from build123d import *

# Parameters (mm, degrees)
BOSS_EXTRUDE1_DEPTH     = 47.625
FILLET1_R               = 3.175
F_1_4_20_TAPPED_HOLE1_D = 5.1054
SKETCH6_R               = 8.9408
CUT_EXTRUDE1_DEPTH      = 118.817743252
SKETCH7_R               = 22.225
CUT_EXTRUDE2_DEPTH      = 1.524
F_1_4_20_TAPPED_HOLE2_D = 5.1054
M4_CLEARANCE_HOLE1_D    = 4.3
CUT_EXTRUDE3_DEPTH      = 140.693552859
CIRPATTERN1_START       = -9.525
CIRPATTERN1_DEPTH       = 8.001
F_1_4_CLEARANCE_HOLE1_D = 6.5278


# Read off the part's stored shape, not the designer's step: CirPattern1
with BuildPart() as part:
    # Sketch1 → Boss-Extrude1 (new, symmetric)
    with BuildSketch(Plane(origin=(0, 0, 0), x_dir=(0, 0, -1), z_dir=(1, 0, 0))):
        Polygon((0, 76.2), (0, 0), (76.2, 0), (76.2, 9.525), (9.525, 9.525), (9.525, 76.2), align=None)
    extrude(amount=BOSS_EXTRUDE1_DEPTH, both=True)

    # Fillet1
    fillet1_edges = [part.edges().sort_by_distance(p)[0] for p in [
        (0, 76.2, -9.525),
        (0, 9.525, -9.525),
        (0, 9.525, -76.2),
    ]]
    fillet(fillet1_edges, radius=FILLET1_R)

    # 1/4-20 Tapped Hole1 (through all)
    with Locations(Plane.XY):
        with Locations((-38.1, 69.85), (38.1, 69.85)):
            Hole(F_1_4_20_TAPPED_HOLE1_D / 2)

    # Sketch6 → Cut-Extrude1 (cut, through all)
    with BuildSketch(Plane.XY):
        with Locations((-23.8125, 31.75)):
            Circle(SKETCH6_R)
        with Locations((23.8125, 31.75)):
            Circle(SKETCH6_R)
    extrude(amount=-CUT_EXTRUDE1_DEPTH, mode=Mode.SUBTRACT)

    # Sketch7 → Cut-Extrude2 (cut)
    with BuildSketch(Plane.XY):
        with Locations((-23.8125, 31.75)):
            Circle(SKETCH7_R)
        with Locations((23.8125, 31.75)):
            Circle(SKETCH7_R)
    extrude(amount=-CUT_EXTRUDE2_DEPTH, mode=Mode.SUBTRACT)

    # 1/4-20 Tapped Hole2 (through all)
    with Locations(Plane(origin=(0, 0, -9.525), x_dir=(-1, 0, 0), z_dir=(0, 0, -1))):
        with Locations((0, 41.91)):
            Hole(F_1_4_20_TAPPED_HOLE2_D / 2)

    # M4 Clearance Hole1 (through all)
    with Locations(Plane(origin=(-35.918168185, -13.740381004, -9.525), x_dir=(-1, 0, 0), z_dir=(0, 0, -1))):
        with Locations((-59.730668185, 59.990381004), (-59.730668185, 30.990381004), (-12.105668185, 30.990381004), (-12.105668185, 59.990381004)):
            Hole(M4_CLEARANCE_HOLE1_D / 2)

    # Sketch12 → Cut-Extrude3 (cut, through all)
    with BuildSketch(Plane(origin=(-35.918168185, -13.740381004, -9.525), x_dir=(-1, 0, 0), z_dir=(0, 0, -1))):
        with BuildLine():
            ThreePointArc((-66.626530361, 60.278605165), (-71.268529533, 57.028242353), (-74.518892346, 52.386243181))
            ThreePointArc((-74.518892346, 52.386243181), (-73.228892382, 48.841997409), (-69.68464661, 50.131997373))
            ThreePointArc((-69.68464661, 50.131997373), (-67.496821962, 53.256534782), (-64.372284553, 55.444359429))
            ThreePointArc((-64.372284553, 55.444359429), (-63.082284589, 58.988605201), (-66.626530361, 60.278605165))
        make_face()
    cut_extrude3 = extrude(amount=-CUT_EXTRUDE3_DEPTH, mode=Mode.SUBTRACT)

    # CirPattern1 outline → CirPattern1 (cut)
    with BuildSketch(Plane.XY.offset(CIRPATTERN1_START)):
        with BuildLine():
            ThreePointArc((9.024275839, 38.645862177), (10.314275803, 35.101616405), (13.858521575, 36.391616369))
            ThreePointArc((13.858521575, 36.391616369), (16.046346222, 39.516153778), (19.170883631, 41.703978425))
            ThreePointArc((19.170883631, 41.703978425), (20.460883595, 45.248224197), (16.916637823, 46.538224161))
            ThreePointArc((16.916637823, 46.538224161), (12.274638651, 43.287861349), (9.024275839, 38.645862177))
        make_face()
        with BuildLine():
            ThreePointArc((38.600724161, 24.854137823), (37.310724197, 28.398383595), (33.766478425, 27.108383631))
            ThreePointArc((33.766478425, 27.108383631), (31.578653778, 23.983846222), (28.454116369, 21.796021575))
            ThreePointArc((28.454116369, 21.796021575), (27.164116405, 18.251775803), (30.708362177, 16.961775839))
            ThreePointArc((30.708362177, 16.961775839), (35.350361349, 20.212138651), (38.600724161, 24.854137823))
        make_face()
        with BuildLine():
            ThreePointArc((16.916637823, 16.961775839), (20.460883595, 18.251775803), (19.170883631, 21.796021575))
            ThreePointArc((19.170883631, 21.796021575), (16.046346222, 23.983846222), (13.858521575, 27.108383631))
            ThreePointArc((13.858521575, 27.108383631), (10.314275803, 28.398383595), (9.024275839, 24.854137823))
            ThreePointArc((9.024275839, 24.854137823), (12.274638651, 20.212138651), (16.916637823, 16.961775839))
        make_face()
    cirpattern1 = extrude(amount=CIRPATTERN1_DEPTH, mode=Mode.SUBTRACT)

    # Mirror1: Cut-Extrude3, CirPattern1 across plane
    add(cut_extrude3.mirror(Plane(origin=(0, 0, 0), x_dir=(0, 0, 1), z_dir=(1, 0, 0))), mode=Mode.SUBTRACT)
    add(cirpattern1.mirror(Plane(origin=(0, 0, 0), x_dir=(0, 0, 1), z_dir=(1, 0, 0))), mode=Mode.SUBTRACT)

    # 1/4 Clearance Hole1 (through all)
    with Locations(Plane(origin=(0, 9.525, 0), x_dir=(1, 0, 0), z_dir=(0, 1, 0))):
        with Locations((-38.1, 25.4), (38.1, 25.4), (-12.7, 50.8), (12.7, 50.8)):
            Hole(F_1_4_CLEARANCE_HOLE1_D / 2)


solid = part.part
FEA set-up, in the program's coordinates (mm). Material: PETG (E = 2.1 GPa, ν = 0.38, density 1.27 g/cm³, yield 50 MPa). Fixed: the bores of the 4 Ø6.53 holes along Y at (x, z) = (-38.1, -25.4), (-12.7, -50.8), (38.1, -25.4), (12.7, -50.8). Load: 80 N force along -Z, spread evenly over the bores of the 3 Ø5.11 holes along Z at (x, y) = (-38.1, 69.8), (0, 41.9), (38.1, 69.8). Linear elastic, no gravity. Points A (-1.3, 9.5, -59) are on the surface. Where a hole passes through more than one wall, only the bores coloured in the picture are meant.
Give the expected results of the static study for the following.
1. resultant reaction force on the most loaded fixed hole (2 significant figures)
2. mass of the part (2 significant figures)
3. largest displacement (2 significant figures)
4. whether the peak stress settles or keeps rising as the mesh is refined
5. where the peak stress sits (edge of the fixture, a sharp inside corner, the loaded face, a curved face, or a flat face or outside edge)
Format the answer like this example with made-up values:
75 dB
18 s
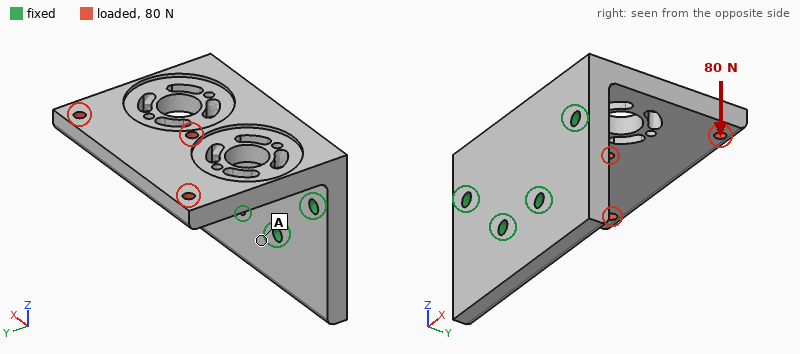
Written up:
45 N
140 g
1.4 mm
keeps rising
a sharp inside corner
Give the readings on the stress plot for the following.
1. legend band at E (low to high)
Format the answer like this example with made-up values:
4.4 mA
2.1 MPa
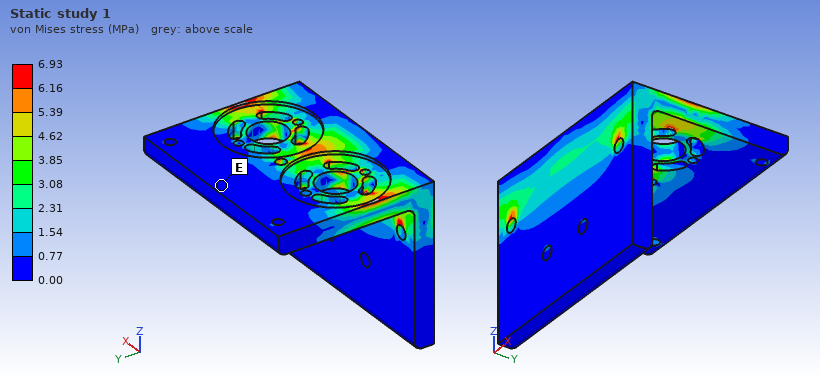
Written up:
0.00 to 0.77 MPa
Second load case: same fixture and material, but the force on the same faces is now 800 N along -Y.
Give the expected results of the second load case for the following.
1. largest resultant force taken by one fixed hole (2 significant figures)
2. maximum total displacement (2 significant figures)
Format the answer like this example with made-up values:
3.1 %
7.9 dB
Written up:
460 N
1.2 mm
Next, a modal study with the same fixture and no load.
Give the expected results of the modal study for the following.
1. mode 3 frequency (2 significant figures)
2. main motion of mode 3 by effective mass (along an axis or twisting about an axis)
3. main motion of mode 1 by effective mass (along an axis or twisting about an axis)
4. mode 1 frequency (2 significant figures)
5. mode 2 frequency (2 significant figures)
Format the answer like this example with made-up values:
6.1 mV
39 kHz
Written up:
850 Hz
along X
along Z
230 Hz
540 Hz
